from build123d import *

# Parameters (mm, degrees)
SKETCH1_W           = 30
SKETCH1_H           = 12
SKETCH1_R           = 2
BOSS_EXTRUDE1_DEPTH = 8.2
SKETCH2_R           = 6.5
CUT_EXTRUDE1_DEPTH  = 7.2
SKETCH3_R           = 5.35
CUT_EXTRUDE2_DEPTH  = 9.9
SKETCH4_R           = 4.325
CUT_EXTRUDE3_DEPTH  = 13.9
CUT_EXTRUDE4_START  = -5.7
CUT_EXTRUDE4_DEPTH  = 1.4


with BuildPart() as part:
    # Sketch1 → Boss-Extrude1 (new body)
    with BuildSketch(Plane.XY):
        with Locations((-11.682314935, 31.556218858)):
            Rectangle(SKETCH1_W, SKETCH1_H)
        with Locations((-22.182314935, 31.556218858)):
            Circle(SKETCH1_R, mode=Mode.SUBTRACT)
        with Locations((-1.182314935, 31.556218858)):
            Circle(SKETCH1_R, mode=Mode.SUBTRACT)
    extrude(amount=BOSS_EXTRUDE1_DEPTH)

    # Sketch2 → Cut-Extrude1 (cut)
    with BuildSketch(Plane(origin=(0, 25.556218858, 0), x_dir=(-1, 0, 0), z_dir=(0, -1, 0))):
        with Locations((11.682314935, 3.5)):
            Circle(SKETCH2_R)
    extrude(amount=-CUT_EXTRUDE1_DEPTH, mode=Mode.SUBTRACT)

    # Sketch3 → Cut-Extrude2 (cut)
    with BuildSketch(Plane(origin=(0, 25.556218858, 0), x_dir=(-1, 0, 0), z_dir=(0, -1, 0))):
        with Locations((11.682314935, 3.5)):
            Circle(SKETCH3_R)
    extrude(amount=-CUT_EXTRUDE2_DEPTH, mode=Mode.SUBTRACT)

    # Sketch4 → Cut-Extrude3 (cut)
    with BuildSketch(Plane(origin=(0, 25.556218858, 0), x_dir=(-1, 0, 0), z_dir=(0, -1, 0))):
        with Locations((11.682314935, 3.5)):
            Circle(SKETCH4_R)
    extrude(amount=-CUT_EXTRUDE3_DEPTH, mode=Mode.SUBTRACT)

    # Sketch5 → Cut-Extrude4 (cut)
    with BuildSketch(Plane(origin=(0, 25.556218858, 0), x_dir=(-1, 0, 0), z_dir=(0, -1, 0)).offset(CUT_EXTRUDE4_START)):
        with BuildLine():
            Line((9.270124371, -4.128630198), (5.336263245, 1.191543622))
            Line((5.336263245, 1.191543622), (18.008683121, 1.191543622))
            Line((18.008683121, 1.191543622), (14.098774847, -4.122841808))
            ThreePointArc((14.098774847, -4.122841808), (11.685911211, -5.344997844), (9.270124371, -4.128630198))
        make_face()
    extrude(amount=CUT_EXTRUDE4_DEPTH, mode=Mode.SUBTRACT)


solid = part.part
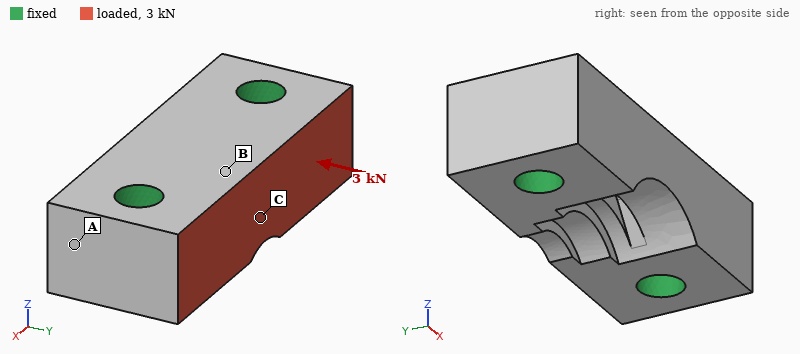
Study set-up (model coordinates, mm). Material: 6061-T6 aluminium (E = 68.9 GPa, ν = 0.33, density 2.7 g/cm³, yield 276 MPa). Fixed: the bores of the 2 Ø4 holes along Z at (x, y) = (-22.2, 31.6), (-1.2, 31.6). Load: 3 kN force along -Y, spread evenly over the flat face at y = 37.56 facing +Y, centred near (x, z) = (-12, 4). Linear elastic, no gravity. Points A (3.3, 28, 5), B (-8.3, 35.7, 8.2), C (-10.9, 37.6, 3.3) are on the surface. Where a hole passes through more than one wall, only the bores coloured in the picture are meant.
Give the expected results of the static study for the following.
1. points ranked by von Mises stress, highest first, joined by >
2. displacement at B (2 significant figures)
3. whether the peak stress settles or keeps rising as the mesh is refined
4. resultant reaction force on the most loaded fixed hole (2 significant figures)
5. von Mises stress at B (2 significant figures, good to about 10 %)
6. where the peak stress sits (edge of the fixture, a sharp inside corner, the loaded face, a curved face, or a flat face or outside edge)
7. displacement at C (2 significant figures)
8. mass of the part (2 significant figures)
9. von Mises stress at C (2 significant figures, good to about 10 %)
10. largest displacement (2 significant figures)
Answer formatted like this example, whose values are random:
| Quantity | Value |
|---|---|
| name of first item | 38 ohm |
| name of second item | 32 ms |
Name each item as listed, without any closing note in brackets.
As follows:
| Quantity | Value |
|---|---|
| points ranked by von Mises stress, highest first, joined by > | C > B > A |
| displacement at B | 3.1 µm |
| whether the peak stress settles or keeps rising as the mesh is refined | keeps rising |
| resultant reaction force on the most loaded fixed hole | 1.5 kN |
| von Mises stress at B | 12 MPa |
| where the peak stress sits | edge of the fixture |
| displacement at C | 4.0 µm |
| mass of the part | 6.8 g |
| von Mises stress at C | 23 MPa |
| largest displacement | 4.8 µm |
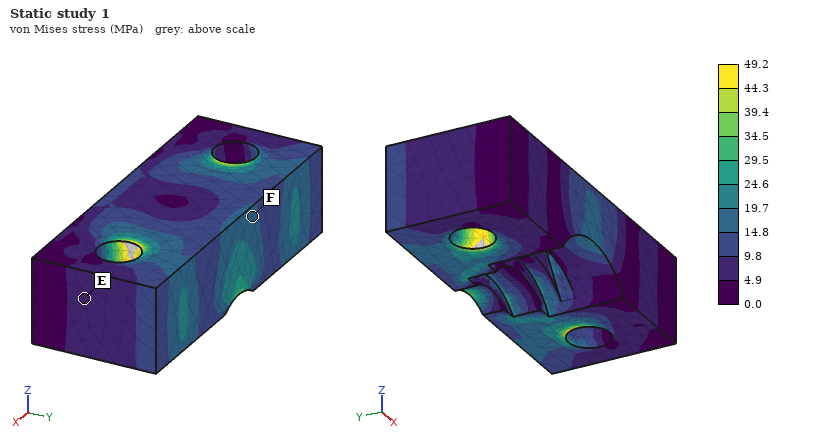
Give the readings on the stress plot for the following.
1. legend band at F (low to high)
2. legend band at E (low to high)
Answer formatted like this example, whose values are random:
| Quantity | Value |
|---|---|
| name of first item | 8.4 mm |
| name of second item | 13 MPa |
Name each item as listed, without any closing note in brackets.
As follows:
| Quantity | Value |
|---|---|
| legend band at F | 14.8 to 19.7 MPa |
| legend band at E | 4.9 to 9.8 MPa |
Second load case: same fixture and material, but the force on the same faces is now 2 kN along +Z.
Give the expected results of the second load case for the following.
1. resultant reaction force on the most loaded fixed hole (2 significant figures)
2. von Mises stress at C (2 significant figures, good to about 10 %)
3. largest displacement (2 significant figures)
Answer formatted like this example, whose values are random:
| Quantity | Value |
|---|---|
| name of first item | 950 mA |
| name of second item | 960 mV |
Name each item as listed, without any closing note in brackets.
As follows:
| Quantity | Value |
|---|---|
| resultant reaction force on the most loaded fixed hole | 1.0 kN |
| von Mises stress at C | 18 MPa |
| largest displacement | 9.6 µm |
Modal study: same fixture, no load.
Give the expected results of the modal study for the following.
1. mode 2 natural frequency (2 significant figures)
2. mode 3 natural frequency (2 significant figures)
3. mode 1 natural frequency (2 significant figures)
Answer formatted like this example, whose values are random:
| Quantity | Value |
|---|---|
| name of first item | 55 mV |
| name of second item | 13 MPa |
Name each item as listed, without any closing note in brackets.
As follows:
| Quantity | Value |
|---|---|
| mode 2 natural frequency | 62 kHz |
| mode 3 natural frequency | 73 kHz |
| mode 1 natural frequency | 61 kHz |
